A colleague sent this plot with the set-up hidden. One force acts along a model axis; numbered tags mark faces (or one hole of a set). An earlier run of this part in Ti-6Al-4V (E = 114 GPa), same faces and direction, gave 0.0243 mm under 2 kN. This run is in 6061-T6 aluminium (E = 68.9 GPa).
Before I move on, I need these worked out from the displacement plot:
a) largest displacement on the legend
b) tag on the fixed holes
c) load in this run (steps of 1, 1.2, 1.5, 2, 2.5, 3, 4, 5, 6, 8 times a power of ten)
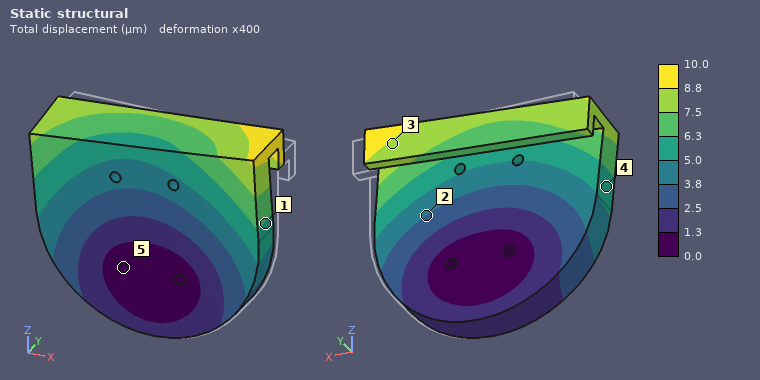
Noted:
10.0 µm
5
500 N
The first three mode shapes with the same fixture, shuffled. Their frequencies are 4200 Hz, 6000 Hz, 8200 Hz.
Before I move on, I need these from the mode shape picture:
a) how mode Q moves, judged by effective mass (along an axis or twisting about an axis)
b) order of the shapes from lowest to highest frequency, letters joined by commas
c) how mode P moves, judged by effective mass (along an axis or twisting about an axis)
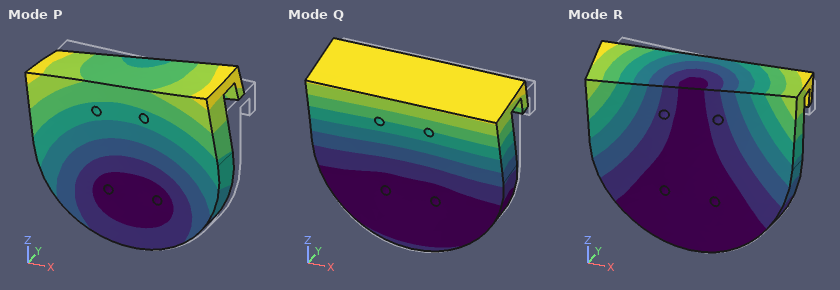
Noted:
along Y
Q, R, P
along X
